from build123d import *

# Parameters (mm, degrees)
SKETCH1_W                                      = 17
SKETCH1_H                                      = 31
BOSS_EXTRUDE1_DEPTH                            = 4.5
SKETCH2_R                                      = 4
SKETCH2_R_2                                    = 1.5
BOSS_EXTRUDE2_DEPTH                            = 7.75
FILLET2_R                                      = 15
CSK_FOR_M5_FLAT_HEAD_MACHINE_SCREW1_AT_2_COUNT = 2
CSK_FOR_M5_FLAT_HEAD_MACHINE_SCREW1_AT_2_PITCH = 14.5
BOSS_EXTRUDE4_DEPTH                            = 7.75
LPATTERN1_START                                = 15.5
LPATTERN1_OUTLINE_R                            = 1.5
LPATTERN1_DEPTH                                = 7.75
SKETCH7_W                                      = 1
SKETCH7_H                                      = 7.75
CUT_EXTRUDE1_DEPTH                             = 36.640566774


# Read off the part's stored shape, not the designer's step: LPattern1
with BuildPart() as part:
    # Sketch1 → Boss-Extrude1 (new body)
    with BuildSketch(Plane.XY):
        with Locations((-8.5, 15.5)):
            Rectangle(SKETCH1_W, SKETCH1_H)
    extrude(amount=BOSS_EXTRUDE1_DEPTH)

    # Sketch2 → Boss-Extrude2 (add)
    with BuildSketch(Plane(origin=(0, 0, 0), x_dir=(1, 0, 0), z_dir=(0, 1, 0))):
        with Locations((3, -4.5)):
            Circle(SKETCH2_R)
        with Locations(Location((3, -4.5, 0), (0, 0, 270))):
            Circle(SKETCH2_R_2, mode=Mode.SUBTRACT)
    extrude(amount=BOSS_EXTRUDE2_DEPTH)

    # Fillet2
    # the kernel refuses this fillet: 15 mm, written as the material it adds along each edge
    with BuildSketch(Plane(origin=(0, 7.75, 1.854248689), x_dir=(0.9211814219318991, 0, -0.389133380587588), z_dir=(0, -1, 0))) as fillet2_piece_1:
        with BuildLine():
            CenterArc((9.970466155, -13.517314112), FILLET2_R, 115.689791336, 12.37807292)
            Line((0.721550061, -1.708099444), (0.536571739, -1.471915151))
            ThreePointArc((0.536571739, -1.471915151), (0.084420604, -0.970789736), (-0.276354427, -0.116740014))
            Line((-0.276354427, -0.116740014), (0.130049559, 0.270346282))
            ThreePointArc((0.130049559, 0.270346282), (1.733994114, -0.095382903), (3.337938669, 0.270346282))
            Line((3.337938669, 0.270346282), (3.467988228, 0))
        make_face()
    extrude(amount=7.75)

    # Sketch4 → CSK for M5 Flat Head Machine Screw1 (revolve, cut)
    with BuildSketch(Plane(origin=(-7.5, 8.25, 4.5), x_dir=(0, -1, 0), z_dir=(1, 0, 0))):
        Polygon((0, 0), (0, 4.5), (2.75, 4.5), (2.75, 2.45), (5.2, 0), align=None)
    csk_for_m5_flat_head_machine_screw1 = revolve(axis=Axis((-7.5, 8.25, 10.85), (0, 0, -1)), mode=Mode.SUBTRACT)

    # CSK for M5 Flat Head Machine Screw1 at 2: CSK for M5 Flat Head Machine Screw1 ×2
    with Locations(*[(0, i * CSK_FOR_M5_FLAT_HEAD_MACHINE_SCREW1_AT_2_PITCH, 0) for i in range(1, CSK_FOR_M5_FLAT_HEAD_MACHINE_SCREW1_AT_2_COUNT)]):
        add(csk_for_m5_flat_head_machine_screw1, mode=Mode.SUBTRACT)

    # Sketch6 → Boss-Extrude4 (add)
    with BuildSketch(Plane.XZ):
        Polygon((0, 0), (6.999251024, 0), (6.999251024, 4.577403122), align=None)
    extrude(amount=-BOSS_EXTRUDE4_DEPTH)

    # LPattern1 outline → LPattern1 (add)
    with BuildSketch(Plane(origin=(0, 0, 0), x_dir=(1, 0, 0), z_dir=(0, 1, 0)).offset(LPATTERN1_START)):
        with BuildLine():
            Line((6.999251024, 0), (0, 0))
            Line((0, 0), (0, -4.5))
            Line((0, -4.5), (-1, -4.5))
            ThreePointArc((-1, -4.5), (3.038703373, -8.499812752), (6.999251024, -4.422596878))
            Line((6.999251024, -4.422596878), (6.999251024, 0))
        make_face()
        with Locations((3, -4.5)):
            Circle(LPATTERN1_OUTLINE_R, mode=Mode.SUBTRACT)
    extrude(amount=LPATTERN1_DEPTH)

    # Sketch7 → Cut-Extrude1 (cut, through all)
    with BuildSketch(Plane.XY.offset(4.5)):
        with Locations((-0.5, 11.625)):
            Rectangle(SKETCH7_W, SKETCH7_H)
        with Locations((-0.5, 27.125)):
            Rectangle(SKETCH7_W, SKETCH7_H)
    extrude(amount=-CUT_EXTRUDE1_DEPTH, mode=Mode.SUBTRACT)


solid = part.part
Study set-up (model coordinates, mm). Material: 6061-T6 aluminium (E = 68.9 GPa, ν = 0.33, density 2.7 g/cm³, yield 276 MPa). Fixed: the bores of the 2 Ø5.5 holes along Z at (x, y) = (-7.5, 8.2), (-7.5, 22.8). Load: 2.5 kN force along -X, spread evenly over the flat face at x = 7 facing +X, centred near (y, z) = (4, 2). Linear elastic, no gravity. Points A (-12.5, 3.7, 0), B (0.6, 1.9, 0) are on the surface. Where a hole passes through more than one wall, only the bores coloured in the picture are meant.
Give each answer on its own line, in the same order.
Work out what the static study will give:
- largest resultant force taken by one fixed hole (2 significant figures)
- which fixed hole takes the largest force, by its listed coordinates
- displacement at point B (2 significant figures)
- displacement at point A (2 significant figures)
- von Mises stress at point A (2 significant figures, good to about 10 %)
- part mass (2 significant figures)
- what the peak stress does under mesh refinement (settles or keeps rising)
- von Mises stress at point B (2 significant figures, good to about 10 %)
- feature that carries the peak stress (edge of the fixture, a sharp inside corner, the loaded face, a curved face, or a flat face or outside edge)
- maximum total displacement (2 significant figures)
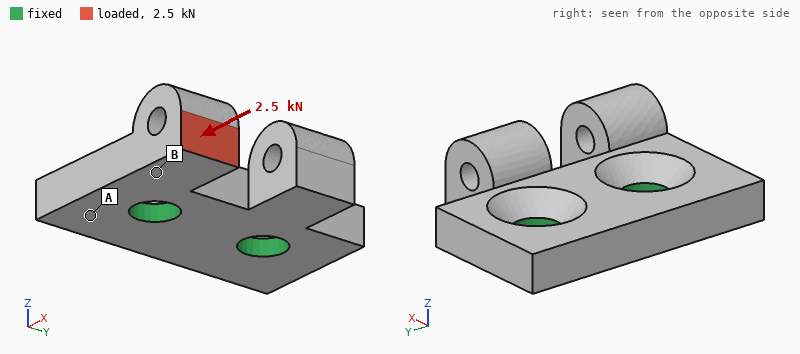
2.8 kN
(-7.5, 8.2)
26 µm
8.9 µm
28 MPa
7.3 g
keeps rising
82 MPa
edge of the fixture
54 µm
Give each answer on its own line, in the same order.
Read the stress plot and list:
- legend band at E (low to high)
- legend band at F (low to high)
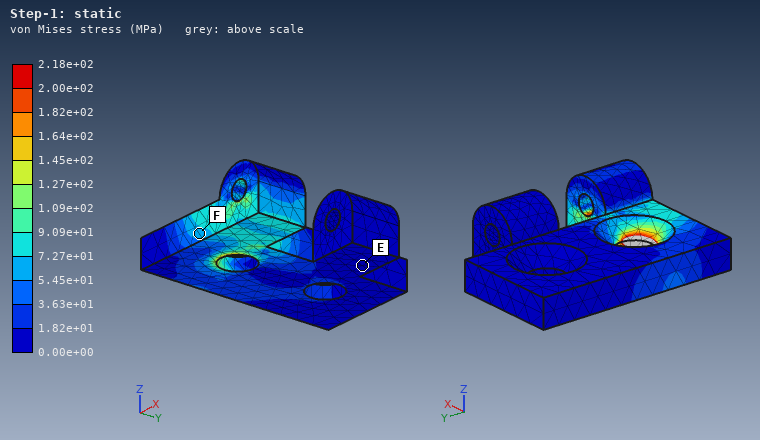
0.00e+00 to 1.82e+01 MPa
5.45e+01 to 7.27e+01 MPa
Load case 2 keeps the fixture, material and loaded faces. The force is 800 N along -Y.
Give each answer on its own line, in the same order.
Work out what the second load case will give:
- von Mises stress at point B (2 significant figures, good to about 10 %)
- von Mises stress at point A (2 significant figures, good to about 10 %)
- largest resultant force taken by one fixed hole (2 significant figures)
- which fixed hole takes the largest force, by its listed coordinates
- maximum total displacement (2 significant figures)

78 MPa
28 MPa
740 N
(-7.5, 8.2)
70 µm
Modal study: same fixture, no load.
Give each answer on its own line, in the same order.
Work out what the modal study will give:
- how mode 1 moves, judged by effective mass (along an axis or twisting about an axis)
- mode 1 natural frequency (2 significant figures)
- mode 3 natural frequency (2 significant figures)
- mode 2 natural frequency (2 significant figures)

along Z
11 kHz
23 kHz
14 kHz
